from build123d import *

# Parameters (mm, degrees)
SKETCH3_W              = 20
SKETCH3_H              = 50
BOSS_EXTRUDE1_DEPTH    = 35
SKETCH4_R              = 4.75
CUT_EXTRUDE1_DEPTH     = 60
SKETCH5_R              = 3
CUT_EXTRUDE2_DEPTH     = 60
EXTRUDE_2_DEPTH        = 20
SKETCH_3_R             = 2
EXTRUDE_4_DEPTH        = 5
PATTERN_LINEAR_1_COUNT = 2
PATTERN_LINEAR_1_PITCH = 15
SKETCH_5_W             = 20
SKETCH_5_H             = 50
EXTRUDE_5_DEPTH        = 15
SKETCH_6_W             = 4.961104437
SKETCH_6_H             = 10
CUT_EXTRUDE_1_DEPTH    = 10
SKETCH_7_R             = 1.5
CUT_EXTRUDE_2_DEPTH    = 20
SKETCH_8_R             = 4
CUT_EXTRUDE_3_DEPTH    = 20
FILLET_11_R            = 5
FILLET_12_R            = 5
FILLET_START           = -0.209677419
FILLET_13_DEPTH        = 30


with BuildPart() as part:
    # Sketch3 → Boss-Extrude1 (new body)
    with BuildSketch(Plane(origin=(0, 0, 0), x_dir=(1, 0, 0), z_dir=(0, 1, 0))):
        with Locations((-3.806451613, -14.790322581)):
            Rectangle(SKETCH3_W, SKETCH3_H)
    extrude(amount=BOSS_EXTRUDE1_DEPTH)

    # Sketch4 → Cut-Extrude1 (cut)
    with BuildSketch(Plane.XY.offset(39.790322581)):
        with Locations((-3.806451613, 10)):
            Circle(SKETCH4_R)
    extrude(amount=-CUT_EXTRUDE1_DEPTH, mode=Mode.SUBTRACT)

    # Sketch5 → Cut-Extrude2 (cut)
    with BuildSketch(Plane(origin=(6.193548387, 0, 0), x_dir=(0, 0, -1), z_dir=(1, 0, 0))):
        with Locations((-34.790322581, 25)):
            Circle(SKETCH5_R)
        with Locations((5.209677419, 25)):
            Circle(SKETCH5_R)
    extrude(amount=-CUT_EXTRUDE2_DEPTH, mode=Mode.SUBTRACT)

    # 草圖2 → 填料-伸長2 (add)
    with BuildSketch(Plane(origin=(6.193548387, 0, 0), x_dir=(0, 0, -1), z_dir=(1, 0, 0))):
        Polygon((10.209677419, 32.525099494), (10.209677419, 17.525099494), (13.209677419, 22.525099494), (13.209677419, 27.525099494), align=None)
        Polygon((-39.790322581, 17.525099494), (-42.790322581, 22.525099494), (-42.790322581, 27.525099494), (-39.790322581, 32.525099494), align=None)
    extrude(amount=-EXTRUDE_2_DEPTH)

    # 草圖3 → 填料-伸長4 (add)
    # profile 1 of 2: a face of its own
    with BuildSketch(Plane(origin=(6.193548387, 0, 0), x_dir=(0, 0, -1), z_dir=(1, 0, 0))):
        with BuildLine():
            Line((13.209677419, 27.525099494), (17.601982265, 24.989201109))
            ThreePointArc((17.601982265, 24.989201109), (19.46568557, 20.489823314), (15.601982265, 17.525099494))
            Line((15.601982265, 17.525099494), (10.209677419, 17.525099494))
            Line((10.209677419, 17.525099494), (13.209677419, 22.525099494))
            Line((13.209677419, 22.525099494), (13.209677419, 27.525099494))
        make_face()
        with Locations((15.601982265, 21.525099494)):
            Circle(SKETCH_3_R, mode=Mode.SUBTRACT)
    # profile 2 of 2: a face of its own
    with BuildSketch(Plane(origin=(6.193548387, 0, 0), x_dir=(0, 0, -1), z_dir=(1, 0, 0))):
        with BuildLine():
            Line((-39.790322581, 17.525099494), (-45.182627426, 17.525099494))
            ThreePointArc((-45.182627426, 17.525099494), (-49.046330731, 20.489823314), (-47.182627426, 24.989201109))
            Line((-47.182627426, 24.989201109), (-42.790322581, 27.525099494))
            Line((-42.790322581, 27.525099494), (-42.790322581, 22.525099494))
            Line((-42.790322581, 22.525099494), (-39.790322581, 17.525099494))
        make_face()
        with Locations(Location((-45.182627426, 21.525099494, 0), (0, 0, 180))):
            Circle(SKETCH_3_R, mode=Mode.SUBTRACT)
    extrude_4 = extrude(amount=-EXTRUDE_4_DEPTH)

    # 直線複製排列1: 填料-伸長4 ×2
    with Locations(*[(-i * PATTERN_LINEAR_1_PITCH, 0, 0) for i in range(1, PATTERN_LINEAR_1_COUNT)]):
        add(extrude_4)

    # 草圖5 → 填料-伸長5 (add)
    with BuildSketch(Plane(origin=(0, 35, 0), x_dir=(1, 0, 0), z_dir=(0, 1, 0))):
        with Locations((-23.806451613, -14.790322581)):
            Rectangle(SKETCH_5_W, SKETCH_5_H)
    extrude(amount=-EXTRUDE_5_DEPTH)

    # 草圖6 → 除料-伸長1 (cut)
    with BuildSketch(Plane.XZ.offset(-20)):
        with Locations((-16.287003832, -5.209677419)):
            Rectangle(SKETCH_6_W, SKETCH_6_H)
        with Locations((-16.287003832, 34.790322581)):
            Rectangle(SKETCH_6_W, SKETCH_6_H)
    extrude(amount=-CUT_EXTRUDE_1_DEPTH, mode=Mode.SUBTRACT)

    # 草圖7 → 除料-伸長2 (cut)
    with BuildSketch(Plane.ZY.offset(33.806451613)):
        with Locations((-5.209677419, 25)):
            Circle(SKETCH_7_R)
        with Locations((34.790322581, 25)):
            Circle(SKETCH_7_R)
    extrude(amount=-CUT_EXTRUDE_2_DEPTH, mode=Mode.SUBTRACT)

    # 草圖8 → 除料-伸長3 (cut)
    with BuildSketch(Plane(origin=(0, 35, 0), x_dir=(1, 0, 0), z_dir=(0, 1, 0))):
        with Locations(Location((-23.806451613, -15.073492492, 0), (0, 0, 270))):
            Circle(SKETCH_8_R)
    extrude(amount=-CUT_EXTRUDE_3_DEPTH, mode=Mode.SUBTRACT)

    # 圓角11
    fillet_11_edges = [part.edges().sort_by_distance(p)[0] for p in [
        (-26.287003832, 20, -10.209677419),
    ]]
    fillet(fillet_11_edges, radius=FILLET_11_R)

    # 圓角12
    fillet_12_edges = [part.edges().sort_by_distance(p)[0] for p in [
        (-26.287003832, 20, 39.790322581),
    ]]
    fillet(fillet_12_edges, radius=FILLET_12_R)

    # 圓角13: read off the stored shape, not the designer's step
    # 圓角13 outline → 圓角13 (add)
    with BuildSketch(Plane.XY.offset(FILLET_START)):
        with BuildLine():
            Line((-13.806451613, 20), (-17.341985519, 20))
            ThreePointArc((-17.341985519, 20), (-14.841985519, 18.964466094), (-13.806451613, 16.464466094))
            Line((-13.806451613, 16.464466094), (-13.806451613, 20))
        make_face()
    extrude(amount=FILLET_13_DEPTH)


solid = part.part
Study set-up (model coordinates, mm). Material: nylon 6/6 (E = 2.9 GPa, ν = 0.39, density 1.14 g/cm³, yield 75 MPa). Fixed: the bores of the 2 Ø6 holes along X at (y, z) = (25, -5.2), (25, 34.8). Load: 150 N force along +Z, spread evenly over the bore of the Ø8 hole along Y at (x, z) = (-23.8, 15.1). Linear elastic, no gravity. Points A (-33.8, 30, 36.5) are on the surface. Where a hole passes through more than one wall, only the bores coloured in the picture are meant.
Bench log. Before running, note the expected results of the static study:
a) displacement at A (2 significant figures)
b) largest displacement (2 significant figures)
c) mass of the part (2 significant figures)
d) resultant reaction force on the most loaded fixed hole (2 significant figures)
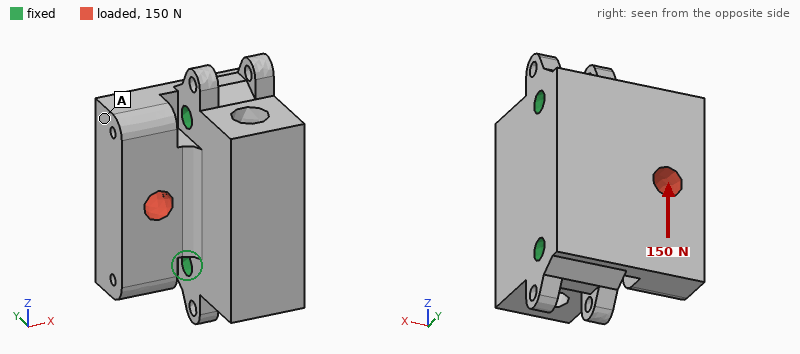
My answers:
8.0 µm
8.6 µm
52 g
98 N
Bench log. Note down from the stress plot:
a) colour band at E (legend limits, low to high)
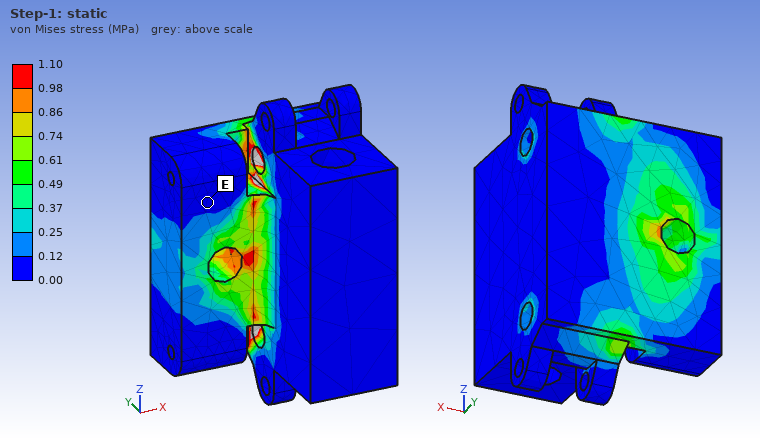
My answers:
0.00 to 0.12 MPa
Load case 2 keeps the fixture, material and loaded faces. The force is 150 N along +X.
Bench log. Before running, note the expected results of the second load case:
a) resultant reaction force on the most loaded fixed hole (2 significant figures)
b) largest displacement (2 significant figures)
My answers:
81 N
6.0 µm
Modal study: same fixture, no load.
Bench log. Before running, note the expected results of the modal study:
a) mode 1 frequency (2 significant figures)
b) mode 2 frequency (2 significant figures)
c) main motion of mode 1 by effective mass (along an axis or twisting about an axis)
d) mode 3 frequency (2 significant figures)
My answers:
3400 Hz
5200 Hz
along Y
5400 Hz
